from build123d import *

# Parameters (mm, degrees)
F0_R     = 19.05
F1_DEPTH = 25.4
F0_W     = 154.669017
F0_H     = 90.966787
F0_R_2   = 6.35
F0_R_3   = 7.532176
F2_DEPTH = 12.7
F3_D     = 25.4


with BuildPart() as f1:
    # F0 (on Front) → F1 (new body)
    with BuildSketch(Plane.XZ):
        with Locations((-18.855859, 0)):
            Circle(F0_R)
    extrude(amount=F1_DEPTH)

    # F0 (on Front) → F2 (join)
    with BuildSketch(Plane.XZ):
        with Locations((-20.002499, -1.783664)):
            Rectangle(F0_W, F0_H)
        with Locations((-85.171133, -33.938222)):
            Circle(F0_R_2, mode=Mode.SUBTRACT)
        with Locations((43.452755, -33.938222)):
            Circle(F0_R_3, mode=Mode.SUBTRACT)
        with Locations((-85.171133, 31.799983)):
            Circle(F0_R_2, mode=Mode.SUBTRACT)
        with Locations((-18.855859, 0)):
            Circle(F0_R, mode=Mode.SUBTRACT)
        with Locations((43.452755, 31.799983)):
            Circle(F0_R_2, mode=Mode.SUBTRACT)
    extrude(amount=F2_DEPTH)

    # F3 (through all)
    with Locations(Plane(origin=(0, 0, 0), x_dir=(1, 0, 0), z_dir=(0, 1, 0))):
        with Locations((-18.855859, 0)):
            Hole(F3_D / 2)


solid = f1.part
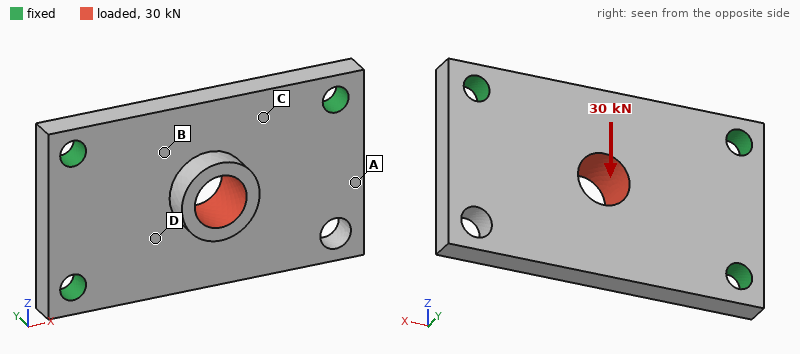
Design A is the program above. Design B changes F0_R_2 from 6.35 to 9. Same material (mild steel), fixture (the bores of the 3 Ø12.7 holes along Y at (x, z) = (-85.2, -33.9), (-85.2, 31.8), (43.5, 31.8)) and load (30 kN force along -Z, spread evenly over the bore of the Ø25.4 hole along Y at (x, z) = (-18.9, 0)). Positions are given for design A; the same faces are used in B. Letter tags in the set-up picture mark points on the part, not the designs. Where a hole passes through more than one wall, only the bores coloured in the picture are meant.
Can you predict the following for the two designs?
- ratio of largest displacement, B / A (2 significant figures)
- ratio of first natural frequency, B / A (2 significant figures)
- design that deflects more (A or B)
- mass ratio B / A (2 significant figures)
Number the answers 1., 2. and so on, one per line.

1. 0.87
2. 1.1
3. A
4. 0.97
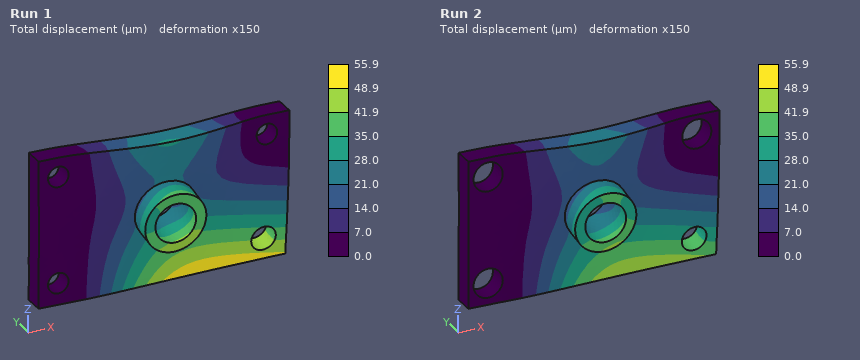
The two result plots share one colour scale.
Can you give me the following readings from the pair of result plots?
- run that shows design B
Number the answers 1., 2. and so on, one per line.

1. Run 2
